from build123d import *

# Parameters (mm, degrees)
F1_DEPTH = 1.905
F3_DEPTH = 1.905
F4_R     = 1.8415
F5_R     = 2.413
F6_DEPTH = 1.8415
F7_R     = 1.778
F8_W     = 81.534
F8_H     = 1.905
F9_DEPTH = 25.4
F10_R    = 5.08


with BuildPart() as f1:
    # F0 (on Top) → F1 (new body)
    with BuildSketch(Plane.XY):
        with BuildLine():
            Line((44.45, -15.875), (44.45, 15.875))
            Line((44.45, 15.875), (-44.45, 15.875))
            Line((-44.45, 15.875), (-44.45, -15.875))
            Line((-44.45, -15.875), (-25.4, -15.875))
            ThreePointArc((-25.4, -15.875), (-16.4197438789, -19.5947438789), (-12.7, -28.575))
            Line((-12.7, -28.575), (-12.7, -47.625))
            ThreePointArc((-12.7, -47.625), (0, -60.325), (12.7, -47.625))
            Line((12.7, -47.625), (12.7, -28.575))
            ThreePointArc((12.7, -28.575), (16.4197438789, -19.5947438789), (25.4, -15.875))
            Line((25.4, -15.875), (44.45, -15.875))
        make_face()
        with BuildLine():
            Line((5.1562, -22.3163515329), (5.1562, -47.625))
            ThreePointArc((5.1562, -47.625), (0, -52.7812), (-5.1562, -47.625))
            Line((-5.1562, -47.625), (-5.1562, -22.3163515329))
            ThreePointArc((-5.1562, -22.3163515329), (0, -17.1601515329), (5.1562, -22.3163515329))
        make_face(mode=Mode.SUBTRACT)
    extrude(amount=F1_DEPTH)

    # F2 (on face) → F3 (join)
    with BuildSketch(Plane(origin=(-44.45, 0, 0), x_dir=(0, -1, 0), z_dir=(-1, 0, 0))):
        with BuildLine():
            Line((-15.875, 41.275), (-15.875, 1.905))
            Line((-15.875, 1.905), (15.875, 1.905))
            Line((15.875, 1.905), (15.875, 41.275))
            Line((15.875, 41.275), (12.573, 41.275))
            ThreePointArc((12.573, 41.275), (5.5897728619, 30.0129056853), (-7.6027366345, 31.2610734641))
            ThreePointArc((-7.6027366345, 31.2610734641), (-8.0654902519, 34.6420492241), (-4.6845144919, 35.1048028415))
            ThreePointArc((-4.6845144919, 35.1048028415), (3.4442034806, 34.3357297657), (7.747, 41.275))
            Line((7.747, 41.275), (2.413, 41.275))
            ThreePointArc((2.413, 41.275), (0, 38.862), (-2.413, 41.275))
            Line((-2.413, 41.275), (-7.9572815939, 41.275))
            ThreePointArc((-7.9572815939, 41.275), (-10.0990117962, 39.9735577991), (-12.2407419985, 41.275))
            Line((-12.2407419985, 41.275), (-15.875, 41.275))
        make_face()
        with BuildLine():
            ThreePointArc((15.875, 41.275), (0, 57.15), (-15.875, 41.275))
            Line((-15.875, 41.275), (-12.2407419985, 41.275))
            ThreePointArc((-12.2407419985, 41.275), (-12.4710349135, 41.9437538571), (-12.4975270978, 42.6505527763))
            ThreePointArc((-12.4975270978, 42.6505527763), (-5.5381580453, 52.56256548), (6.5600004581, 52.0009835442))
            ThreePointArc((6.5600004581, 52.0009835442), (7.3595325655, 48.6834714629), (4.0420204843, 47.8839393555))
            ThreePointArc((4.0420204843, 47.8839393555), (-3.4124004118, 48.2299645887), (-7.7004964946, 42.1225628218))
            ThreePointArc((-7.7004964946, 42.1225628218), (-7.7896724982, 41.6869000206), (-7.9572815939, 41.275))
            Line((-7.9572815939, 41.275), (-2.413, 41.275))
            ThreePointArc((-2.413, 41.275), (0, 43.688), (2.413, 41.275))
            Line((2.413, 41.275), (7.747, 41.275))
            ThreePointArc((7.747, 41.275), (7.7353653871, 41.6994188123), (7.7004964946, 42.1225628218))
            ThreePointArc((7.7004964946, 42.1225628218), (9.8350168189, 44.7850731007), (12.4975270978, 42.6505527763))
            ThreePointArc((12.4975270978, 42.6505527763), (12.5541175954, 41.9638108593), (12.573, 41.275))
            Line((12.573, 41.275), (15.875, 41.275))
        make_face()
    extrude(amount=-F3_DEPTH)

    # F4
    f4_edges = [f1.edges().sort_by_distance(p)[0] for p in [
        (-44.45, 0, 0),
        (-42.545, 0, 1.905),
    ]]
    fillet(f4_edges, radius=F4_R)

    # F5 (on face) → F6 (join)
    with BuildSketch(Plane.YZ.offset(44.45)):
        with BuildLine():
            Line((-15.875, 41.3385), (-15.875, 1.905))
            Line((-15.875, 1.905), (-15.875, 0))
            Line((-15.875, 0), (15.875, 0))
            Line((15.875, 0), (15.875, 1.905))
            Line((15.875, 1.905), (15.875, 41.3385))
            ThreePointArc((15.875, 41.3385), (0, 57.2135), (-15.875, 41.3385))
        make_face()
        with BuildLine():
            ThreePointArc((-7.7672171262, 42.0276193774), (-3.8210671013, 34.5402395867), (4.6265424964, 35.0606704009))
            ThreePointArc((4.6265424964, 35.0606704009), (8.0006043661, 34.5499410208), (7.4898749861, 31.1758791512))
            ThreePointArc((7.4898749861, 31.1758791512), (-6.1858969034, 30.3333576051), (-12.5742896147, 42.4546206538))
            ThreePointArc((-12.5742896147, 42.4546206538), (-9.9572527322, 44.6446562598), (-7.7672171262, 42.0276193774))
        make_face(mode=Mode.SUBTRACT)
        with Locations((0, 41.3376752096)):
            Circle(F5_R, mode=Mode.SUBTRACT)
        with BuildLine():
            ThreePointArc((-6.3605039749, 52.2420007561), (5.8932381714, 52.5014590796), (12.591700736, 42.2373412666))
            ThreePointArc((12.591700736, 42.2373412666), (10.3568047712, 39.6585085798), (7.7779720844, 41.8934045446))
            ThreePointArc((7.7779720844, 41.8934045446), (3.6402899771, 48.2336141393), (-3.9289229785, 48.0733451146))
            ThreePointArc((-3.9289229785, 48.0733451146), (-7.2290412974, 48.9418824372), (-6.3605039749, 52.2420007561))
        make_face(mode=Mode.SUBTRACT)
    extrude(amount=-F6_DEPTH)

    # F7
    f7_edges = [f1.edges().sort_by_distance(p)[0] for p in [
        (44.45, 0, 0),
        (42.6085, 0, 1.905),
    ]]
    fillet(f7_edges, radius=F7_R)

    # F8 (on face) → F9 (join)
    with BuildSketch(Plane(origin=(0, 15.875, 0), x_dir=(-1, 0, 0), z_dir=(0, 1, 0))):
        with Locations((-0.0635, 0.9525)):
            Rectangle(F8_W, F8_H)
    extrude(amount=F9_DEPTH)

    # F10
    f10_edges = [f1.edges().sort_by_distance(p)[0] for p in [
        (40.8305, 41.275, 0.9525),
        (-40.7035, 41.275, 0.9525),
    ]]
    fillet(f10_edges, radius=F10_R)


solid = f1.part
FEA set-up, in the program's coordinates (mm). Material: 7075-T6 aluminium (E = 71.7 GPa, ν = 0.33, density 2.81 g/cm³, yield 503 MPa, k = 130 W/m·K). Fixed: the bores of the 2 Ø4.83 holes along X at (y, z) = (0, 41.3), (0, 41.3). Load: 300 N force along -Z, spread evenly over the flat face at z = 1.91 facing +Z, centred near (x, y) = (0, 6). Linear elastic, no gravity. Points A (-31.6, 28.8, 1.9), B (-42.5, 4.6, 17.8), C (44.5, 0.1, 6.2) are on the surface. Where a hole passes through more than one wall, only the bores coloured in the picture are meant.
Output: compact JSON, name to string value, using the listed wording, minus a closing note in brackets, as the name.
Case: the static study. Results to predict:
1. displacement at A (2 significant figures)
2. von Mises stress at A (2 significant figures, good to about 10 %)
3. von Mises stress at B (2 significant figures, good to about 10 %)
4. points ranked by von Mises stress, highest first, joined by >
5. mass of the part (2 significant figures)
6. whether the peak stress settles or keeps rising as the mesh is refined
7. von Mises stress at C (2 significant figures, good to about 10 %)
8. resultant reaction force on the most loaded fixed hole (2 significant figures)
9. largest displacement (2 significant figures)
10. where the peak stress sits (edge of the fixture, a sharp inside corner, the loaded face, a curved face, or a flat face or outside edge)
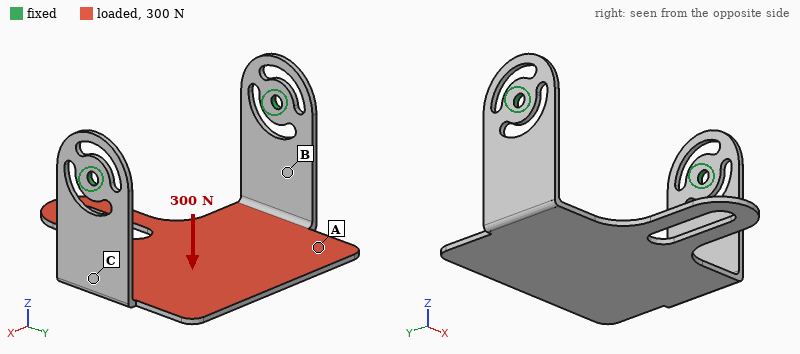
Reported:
{"displacement at A": "0.37 mm", "von Mises stress at A": "23 MPa", "von Mises stress at B": "44 MPa", "points ranked by von Mises stress, highest first, joined by >": "C > B > A", "mass of the part": "45 g", "whether the peak stress settles or keeps rising as the mesh is refined": "keeps rising", "von Mises stress at C": "65 MPa", "resultant reaction force on the most loaded fixed hole": "160 N", "largest displacement": "1.8 mm", "where the peak stress sits": "a sharp inside corner"}
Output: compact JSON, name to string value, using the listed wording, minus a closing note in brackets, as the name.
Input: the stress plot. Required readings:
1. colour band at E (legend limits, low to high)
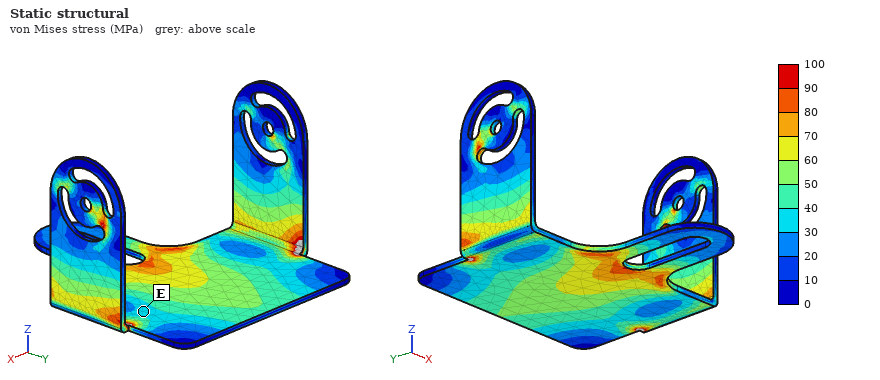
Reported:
{"colour band at E": "30 to 40 MPa"}
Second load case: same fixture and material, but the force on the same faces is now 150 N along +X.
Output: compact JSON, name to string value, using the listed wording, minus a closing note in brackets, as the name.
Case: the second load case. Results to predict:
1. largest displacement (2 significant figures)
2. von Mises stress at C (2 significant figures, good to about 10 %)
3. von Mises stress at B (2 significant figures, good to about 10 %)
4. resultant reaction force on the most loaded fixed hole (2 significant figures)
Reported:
{"largest displacement": "0.99 mm", "von Mises stress at C": "71 MPa", "von Mises stress at B": "35 MPa", "resultant reaction force on the most loaded fixed hole": "86 N"}
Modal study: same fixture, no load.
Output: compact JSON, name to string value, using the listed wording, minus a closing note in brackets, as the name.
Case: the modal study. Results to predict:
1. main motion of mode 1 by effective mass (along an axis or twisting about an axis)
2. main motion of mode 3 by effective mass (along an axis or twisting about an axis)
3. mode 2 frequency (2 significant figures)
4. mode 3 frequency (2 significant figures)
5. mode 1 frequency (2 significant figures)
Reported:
{"main motion of mode 1 by effective mass": "along X", "main motion of mode 3 by effective mass": "along Z", "mode 2 frequency": "490 Hz", "mode 3 frequency": "680 Hz", "mode 1 frequency": "330 Hz"}
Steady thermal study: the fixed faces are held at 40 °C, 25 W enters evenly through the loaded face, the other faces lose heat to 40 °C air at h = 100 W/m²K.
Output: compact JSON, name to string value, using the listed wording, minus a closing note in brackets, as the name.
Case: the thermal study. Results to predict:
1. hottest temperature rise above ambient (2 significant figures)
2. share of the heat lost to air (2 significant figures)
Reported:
{"hottest temperature rise above ambient": "29 K", "share of the heat lost to air": "91 %"}
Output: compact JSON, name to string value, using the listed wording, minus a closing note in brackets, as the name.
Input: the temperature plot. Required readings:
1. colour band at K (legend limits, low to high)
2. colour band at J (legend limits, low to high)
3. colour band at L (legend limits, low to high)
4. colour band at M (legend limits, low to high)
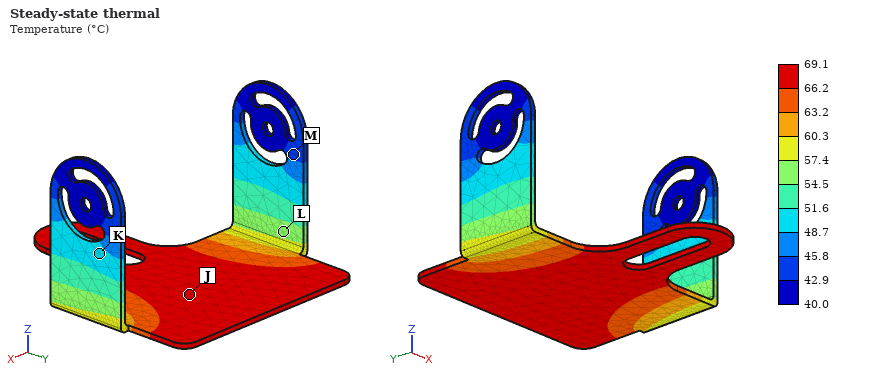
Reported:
{"colour band at K": "48.7 to 51.6 °C", "colour band at J": "66.2 to 69.1 °C", "colour band at L": "54.5 to 57.4 °C", "colour band at M": "42.9 to 45.8 °C"}
